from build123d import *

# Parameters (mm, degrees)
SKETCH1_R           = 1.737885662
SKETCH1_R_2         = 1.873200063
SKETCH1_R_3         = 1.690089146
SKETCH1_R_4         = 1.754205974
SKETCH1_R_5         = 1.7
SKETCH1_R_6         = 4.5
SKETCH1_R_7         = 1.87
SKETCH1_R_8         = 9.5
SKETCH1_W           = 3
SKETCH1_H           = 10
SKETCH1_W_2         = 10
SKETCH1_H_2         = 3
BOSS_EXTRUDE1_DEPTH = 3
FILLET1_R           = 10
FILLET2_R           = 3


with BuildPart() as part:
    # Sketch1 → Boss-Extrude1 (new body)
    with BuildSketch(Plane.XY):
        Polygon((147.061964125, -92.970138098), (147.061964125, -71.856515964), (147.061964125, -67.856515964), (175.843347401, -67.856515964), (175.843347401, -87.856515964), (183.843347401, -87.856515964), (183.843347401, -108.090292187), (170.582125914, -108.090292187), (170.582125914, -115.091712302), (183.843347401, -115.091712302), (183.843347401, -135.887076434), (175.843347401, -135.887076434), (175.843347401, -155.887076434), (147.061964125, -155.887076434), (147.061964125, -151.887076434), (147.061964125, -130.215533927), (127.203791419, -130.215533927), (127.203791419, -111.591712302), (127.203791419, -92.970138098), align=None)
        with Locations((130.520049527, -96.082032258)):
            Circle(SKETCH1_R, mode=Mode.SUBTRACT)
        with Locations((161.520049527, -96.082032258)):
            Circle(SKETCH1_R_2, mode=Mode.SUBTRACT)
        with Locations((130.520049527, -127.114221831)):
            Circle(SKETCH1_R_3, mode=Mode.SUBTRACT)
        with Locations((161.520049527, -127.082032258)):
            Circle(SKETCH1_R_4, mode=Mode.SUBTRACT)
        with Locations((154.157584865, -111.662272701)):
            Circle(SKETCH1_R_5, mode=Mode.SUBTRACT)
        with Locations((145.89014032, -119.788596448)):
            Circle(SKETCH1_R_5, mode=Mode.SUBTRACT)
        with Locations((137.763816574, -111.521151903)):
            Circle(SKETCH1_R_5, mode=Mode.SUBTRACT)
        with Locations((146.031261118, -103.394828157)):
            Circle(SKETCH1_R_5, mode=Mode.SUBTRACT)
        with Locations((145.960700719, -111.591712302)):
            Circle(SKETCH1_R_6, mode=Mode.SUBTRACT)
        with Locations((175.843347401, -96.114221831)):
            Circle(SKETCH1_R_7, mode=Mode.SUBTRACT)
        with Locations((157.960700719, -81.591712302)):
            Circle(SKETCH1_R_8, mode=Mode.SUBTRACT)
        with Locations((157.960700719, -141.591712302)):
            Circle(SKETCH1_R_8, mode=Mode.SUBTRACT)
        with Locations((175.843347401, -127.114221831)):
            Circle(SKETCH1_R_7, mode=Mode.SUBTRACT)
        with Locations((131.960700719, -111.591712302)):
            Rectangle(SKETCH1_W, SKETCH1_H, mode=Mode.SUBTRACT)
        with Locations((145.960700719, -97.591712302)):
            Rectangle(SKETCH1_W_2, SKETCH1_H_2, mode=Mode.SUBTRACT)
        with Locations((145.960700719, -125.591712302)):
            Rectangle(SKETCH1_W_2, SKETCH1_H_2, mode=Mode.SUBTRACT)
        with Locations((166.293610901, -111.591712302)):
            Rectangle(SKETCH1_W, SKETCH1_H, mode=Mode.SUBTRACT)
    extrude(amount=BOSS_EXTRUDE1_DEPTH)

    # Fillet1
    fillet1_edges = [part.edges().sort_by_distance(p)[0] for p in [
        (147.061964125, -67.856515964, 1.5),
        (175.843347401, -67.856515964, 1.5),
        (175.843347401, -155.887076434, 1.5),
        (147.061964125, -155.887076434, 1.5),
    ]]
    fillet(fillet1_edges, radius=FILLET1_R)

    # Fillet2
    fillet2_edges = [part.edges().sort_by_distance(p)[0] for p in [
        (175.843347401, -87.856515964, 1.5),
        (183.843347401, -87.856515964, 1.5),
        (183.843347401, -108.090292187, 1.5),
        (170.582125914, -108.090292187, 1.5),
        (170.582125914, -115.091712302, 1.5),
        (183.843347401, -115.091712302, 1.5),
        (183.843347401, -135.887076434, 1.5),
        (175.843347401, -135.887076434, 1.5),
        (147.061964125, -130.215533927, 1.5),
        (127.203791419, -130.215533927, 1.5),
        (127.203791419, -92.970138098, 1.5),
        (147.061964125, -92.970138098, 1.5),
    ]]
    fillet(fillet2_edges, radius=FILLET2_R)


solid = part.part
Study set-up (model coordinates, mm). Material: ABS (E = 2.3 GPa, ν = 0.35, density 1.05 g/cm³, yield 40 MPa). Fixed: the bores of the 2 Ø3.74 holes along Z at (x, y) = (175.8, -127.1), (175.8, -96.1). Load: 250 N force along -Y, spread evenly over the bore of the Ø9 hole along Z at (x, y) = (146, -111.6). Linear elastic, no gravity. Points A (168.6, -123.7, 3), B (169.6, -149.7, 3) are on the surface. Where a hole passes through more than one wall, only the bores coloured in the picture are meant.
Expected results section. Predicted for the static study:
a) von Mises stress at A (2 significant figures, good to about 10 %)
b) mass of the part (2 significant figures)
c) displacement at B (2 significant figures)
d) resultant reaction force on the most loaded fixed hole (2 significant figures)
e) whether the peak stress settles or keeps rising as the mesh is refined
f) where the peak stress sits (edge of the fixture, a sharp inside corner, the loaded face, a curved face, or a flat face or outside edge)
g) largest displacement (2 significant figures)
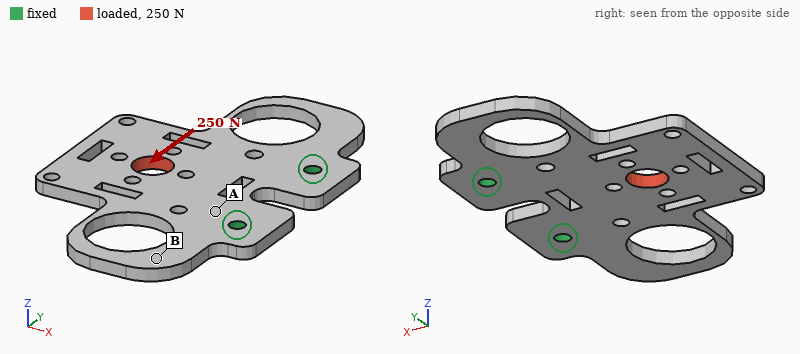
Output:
6.8 MPa
8.3 g
0.14 mm
240 N
keeps rising
edge of the fixture
0.28 mm
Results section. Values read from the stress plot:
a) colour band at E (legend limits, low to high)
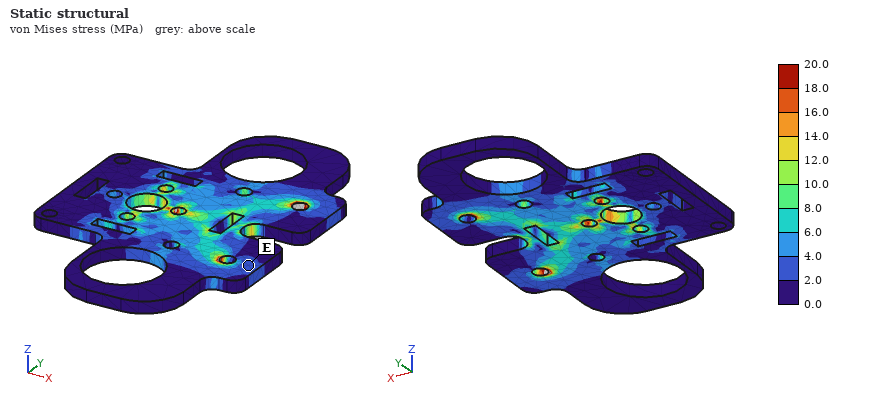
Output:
2.0 to 4.0 MPa
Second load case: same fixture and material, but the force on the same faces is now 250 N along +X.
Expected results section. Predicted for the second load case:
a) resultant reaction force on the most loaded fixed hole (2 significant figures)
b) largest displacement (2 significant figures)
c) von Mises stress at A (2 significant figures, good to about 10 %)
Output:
130 N
66 µm
3.7 MPa
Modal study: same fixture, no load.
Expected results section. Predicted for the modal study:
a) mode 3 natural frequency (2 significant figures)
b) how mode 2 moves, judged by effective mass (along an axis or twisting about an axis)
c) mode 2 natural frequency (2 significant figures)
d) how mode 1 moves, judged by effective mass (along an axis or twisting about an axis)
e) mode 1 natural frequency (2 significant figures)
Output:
790 Hz
twisting about X
680 Hz
along Z
330 Hz
